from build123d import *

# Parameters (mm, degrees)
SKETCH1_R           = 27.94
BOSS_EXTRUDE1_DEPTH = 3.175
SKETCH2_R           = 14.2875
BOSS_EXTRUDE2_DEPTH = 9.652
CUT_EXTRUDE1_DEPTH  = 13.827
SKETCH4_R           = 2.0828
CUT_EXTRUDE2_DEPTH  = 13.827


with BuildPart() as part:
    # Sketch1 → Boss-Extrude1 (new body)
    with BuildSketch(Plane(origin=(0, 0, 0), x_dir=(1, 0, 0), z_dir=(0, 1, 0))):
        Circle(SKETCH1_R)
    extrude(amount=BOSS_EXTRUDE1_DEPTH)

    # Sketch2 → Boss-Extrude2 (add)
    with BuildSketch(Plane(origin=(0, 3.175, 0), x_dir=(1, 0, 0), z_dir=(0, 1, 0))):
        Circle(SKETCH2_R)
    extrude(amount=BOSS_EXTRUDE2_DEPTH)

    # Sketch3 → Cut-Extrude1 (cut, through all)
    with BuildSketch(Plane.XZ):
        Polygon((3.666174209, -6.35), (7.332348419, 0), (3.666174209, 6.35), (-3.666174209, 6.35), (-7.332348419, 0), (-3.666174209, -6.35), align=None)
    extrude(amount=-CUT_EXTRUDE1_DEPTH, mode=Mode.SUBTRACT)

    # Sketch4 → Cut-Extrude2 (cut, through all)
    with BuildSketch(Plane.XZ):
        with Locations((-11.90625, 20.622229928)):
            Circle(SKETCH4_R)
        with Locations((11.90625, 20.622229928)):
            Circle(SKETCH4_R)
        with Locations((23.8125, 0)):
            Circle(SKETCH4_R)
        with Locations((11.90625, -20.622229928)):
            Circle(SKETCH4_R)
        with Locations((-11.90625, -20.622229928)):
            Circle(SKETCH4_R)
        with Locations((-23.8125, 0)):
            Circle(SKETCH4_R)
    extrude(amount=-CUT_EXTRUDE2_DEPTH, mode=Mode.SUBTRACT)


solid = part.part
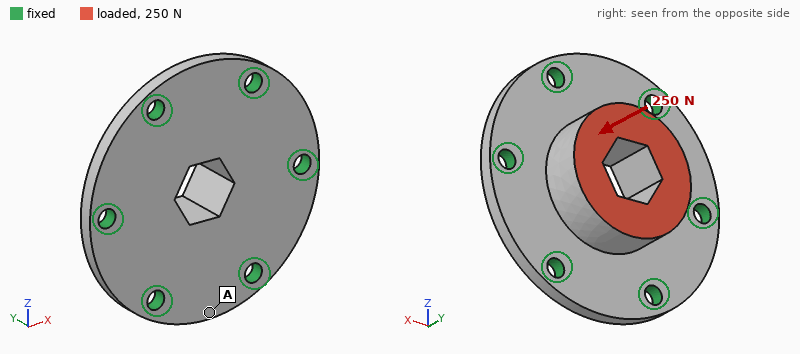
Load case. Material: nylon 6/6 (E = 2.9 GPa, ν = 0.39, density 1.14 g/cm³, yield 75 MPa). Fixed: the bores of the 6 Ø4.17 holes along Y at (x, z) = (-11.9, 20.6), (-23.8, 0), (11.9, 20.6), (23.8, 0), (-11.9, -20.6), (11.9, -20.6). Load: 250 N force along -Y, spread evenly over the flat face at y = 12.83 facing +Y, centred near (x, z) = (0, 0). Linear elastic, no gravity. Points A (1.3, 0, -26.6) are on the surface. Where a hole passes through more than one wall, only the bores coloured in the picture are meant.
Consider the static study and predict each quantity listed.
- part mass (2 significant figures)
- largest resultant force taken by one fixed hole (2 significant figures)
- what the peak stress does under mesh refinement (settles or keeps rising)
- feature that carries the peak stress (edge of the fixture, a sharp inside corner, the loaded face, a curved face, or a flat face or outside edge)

14 g
47 N
keeps rising
edge of the fixture
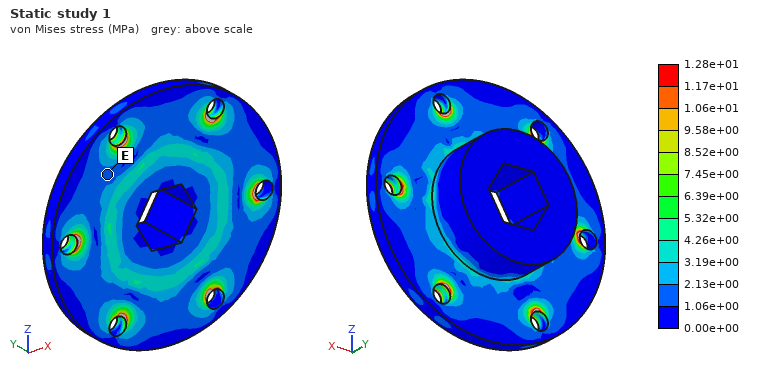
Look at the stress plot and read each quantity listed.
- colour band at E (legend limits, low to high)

1.06e+00 to 2.13e+00 MPa
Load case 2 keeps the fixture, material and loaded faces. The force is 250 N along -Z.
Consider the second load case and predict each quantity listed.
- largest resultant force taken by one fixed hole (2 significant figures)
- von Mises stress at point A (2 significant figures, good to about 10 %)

68 N
1.6 MPa
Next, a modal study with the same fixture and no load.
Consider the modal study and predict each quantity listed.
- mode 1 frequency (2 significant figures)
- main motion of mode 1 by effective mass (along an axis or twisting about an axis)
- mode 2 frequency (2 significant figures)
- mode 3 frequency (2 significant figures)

4200 Hz
along Y
5600 Hz
5600 Hz
